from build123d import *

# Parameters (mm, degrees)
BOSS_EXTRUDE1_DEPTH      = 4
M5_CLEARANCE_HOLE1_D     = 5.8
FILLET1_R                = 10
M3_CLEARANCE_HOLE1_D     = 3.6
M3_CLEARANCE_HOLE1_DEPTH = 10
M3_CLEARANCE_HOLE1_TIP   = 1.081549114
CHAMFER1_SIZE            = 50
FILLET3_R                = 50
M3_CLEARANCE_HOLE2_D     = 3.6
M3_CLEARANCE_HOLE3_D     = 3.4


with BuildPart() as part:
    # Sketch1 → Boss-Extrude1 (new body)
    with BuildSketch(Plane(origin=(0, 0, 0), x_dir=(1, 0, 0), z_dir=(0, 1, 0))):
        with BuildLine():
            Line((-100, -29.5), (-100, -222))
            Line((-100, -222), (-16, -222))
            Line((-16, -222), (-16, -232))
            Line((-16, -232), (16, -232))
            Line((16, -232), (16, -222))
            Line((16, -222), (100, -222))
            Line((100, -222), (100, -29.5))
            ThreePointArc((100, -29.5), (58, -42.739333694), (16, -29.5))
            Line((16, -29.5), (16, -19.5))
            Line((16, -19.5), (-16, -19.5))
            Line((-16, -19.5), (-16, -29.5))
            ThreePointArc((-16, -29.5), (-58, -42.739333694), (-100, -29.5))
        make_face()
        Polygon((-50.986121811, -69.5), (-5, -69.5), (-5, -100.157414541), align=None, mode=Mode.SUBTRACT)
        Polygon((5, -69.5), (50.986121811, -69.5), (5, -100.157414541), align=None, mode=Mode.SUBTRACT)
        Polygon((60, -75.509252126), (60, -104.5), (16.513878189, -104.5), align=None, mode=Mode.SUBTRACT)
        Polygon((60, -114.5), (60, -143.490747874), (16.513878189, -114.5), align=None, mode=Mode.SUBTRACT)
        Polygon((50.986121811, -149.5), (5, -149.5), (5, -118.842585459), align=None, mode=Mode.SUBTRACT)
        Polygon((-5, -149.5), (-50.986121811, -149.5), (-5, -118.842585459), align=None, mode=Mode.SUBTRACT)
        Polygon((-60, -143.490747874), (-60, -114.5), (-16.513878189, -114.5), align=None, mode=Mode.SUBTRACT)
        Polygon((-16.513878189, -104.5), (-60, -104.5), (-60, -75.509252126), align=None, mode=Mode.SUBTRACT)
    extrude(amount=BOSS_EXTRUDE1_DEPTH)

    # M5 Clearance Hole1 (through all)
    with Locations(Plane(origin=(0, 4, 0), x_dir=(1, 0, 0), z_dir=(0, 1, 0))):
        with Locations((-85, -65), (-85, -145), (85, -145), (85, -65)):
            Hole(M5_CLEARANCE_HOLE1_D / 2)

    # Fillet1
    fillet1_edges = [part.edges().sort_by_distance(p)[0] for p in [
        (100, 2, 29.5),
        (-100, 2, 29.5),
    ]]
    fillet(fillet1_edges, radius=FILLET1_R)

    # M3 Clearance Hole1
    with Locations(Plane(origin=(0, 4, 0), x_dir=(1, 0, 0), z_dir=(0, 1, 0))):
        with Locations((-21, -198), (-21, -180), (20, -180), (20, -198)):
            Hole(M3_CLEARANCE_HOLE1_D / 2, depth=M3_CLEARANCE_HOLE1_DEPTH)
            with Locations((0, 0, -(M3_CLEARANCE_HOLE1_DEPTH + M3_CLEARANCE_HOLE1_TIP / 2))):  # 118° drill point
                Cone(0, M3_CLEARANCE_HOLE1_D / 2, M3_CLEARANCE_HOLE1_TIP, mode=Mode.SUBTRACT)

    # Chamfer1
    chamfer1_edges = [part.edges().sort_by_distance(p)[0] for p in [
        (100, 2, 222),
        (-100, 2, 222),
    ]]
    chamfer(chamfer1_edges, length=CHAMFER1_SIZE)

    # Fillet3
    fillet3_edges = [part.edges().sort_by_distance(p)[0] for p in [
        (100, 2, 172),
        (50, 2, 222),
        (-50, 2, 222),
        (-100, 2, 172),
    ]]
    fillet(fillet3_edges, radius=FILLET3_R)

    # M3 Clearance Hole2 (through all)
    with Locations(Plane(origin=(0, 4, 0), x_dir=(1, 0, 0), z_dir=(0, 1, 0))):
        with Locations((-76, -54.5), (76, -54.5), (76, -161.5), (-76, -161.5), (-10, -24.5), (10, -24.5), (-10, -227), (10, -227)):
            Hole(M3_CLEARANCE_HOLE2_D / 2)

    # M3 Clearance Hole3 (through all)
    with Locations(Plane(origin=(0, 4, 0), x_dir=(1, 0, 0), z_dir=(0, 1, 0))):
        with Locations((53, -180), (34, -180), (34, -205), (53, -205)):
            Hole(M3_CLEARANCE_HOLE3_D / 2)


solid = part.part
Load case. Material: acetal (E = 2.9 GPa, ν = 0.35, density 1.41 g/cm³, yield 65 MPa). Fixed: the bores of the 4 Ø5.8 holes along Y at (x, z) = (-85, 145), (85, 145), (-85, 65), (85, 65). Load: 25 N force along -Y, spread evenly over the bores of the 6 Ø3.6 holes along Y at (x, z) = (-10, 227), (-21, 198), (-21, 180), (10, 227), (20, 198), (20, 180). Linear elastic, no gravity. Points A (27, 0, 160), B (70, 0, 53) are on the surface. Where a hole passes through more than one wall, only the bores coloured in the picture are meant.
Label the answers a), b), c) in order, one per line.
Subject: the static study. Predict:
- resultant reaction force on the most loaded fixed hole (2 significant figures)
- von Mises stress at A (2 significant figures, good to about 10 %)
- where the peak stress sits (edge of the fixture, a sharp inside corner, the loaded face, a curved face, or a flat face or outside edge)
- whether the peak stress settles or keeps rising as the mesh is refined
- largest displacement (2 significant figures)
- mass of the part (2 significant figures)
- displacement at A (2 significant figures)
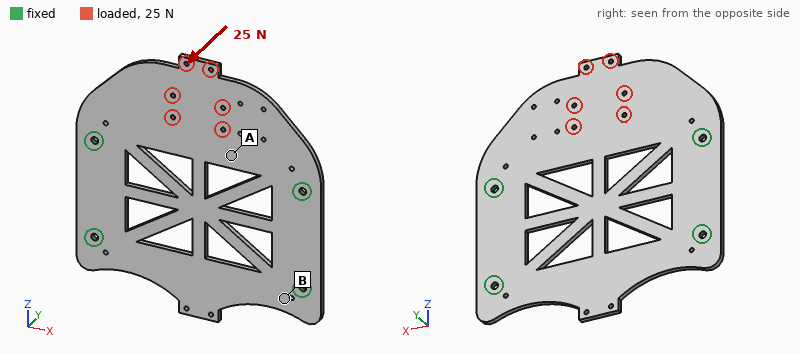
a) 15 N
b) 1.6 MPa
c) edge of the fixture
d) keeps rising
e) 3.1 mm
f) 160 g
g) 0.68 mm
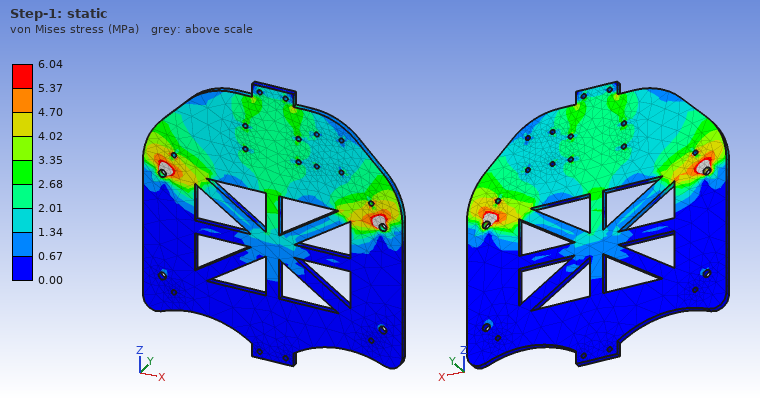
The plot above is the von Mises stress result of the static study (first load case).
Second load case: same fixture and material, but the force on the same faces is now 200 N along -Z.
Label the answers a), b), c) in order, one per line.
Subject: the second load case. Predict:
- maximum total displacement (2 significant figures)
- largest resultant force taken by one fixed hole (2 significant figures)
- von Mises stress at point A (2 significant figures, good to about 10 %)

a) 37 µm
b) 85 N
c) 0.33 MPa
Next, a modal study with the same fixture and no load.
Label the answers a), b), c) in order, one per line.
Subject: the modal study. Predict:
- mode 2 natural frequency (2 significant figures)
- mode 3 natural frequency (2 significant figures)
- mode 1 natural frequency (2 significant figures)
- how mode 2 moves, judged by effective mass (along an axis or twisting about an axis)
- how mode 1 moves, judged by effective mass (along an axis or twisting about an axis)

a) 180 Hz
b) 250 Hz
c) 100 Hz
d) along Y
e) along Y
